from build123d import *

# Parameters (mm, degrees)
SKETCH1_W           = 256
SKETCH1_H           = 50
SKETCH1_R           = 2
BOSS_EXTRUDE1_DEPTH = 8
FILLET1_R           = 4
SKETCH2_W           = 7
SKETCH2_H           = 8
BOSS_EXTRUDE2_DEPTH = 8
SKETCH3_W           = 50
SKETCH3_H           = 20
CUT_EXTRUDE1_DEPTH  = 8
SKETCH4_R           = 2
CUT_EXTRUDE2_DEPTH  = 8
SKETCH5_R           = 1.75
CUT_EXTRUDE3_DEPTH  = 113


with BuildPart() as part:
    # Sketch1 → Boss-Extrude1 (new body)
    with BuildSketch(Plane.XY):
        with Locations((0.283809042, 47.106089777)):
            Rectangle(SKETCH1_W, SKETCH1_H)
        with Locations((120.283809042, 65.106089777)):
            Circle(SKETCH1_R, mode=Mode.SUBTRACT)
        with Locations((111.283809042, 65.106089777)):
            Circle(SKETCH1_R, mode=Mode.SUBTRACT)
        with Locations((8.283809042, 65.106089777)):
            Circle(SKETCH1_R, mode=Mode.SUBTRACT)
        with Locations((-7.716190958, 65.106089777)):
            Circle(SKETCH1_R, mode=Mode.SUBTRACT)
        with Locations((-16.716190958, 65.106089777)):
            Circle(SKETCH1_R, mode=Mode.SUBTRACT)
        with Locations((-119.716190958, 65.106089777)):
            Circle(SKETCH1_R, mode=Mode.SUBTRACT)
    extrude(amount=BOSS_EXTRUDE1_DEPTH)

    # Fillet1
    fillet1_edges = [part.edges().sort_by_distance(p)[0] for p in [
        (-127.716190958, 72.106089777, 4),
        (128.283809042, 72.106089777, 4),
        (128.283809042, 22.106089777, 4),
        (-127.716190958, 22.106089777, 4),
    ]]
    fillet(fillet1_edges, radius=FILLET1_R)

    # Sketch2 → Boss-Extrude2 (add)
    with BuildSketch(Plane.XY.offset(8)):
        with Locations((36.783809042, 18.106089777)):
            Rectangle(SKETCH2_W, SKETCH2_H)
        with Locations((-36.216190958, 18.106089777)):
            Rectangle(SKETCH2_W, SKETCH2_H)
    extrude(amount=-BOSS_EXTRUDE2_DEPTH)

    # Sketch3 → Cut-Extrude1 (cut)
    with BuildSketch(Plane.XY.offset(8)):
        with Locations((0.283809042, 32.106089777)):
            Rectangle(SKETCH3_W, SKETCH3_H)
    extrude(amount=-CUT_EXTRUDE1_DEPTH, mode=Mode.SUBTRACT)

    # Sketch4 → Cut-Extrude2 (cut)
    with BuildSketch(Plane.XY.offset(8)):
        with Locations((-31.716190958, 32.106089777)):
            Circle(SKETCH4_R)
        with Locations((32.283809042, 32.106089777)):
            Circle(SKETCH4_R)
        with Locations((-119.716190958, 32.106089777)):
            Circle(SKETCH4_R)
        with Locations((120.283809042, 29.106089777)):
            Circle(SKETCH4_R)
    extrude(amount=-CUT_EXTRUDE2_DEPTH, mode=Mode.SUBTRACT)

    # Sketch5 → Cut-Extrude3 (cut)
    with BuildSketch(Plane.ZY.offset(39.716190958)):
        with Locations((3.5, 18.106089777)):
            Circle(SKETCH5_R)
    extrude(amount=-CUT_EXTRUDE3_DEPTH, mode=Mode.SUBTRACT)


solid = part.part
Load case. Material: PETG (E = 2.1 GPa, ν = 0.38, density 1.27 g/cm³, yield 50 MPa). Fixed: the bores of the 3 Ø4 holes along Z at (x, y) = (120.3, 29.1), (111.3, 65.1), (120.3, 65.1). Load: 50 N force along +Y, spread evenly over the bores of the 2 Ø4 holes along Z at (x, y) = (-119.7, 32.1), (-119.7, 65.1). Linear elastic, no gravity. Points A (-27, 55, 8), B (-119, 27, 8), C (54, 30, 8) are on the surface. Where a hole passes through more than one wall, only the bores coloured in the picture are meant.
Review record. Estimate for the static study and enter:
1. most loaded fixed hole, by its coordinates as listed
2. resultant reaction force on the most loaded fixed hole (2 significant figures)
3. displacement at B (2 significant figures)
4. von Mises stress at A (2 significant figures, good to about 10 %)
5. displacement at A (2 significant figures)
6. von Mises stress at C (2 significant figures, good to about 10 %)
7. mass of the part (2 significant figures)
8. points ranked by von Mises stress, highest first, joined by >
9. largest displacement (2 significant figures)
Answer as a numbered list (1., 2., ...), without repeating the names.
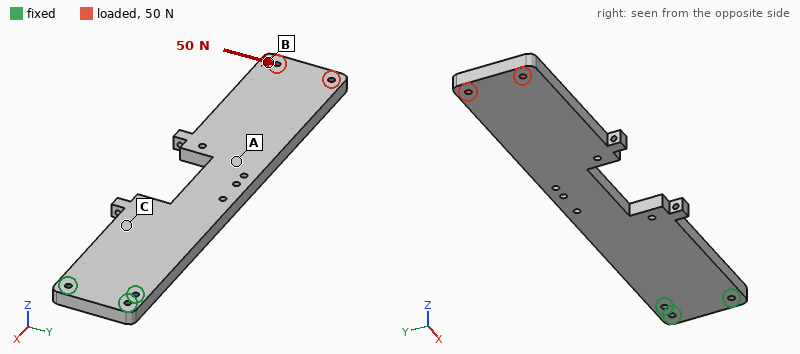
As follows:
1. (120.3, 29.1)
2. 300 N
3. 2.6 mm
4. 1.1 MPa
5. 0.90 mm
6. 1.8 MPa
7. 120 g
8. C > A > B
9. 2.7 mm
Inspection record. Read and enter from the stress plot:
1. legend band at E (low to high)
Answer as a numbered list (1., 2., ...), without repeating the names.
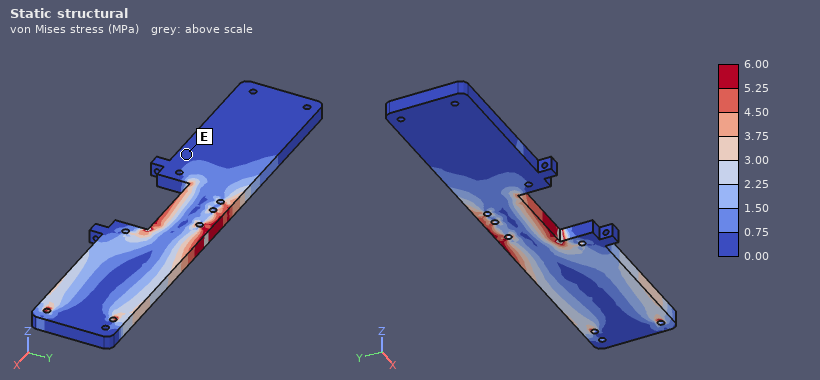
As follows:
1. 0.00 to 0.75 MPa
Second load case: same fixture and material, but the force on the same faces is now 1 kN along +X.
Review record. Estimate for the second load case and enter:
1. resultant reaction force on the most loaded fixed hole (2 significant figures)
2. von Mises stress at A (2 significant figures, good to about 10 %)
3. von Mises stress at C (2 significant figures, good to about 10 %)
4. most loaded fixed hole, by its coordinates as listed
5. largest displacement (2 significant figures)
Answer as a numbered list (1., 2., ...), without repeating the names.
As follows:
1. 460 N
2. 4.1 MPa
3. 2.1 MPa
4. (120.3, 29.1)
5. 2.2 mm
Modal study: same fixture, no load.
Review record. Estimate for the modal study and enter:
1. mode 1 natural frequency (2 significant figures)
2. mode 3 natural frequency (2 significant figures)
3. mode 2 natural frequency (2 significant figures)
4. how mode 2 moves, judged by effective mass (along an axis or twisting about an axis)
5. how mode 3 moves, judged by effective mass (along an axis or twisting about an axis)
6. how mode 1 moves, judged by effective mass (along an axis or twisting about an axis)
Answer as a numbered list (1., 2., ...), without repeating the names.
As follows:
1. 27 Hz
2. 170 Hz
3. 130 Hz
4. along Y
5. along Z
6. along Z
